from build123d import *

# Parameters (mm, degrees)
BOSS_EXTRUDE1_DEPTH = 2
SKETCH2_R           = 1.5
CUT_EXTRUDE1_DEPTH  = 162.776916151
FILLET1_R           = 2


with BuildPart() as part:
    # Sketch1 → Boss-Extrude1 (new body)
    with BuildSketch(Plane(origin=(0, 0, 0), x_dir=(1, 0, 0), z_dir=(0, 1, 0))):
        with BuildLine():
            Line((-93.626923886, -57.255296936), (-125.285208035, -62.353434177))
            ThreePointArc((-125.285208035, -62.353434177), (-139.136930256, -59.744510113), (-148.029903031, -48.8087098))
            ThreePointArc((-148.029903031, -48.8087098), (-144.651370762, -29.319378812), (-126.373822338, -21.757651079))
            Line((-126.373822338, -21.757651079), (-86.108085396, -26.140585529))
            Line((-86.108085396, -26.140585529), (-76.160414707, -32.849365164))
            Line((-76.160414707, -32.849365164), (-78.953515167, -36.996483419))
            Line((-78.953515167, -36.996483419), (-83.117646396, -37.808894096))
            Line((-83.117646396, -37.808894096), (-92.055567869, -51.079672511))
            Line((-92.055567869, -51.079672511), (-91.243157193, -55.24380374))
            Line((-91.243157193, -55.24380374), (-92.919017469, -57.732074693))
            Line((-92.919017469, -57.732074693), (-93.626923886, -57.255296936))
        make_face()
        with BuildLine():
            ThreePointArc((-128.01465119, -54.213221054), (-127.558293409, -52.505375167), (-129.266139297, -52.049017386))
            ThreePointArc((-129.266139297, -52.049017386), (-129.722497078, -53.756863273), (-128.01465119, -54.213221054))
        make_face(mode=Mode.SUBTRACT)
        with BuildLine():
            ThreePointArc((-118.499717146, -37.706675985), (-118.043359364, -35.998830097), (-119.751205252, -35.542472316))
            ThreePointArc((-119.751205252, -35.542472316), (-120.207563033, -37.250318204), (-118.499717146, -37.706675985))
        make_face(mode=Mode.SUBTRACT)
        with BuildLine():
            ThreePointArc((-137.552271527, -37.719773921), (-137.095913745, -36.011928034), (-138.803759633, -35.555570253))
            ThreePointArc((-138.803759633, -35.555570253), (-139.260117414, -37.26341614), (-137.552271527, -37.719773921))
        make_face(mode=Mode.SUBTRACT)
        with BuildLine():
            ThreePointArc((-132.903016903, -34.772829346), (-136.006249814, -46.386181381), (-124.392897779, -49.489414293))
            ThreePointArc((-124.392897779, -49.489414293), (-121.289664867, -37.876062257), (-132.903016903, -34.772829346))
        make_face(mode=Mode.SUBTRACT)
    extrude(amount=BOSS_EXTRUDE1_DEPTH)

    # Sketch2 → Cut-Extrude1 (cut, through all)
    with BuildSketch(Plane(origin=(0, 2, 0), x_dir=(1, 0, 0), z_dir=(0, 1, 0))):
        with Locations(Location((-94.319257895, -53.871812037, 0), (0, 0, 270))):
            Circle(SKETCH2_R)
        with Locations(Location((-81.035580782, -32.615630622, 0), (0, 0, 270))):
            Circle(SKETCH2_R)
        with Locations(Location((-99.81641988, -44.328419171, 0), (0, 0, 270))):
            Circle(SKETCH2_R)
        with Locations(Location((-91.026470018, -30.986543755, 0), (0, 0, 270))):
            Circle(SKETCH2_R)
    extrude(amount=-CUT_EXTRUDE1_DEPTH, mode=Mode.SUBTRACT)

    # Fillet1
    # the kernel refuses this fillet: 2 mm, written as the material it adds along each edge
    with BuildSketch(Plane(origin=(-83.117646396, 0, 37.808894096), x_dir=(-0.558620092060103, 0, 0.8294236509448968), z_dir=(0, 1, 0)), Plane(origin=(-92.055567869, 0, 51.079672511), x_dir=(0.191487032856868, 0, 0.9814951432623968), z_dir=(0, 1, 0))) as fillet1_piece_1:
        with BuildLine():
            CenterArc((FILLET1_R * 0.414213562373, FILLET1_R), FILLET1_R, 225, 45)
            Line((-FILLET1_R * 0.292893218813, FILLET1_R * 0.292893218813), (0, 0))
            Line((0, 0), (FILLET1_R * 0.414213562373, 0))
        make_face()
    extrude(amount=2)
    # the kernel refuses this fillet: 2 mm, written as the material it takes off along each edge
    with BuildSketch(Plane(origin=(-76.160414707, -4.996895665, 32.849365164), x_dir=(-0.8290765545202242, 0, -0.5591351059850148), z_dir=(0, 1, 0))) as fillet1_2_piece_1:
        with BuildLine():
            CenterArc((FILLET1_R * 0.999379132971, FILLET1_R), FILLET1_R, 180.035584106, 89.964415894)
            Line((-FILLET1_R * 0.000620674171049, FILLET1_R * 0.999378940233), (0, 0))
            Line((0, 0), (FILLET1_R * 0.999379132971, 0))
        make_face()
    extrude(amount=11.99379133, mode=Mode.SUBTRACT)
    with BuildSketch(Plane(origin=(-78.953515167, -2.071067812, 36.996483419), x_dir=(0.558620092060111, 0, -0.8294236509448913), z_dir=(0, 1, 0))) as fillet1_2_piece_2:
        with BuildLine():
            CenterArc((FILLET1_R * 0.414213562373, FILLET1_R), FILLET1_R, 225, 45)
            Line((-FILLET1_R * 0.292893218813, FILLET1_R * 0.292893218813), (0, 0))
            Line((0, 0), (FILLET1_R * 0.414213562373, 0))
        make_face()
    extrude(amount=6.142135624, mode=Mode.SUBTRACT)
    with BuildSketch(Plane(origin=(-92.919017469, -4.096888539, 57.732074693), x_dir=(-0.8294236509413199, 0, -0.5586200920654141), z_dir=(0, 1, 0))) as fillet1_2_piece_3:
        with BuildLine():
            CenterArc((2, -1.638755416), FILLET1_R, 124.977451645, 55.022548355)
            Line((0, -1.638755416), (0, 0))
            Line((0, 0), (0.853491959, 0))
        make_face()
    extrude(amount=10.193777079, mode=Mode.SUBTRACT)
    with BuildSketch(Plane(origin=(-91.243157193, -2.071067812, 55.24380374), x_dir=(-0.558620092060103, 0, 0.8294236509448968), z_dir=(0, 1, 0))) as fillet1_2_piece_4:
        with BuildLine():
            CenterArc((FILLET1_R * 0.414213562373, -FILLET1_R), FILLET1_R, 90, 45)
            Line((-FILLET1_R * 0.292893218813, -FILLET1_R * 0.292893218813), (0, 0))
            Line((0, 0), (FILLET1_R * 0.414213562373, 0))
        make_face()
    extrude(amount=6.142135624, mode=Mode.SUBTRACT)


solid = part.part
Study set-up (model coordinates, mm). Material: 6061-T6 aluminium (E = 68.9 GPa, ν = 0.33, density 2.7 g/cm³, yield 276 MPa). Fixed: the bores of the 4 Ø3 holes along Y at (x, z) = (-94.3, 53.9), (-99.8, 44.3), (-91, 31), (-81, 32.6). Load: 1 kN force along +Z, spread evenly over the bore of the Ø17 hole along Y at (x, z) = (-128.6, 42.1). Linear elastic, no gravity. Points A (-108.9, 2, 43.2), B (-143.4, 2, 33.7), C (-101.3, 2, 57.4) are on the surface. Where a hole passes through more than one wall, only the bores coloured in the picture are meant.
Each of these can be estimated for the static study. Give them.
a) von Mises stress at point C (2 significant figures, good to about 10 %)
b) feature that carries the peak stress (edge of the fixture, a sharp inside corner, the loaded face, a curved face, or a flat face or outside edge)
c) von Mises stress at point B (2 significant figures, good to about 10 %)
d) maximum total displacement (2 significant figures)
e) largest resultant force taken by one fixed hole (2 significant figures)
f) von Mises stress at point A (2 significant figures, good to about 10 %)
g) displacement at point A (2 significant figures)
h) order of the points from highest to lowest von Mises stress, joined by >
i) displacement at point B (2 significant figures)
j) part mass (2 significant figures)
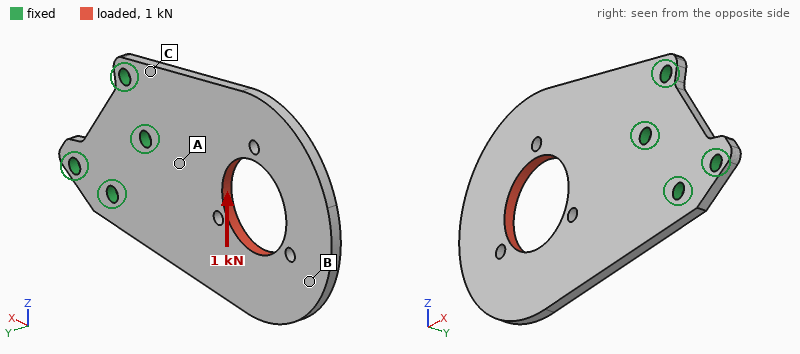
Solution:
72 MPa
edge of the fixture
9.5 MPa
0.10 mm
1.1 kN
47 MPa
0.016 mm
C > A > B
0.097 mm
10 g
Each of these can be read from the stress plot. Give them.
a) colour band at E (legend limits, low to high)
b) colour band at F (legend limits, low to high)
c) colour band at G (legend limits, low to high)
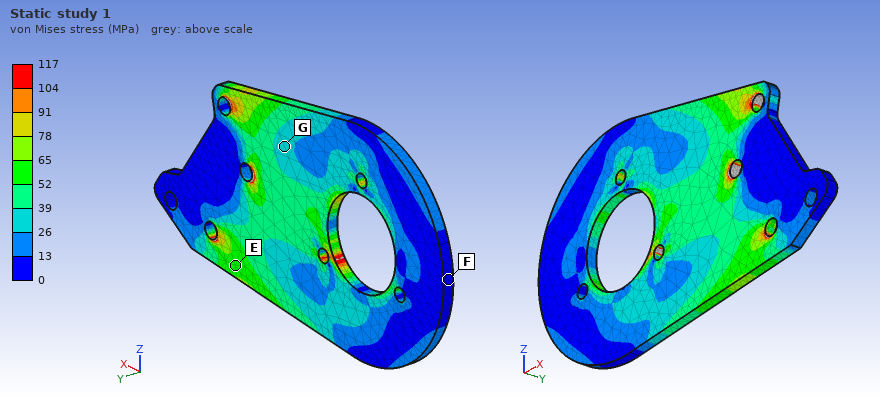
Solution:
52 to 65 MPa
0 to 13 MPa
26 to 39 MPa
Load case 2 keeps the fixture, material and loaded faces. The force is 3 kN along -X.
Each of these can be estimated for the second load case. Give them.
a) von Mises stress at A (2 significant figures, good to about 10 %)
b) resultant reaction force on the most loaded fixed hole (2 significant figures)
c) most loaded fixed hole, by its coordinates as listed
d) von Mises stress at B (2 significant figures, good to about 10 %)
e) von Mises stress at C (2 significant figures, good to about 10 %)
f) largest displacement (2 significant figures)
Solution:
45 MPa
1.2 kN
(-99.8, 44.3)
27 MPa
48 MPa
42 µm
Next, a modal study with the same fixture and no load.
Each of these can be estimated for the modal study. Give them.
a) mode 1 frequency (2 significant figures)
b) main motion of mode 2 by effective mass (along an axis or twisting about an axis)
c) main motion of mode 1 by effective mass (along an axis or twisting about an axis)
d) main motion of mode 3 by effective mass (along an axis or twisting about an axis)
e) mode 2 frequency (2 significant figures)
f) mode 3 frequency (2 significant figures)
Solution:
740 Hz
twisting about X
along Y
along Y
1800 Hz
3600 Hz
